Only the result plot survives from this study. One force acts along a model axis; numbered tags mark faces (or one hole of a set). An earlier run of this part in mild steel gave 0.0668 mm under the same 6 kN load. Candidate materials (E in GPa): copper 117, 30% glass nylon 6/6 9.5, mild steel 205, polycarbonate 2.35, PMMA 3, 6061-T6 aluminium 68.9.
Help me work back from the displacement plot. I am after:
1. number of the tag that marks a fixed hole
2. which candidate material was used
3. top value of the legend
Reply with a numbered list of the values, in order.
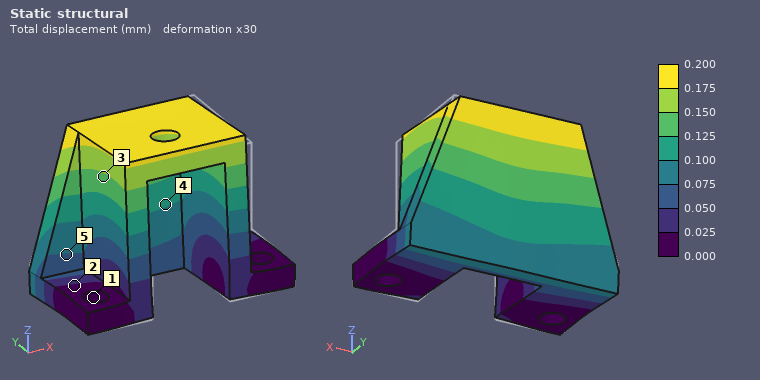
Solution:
1. 1
2. 6061-T6 aluminium
3. 0.200 mm
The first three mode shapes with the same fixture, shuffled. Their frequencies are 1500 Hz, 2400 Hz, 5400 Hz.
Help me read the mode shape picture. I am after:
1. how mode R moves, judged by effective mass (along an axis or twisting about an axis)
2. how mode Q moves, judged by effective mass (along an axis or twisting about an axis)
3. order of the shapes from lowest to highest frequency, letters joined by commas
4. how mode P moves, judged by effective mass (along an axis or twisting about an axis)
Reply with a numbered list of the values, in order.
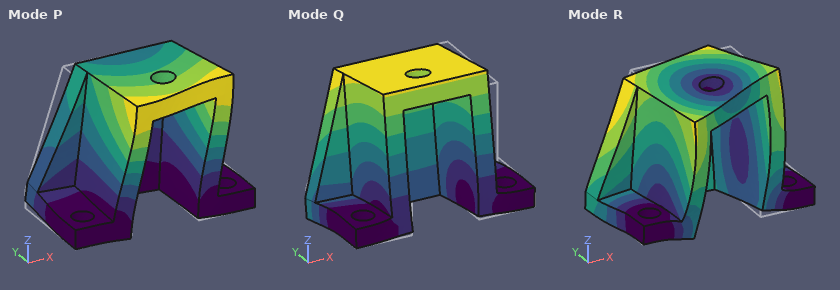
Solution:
1. along X
2. along Y
3. Q, P, R
4. along X
